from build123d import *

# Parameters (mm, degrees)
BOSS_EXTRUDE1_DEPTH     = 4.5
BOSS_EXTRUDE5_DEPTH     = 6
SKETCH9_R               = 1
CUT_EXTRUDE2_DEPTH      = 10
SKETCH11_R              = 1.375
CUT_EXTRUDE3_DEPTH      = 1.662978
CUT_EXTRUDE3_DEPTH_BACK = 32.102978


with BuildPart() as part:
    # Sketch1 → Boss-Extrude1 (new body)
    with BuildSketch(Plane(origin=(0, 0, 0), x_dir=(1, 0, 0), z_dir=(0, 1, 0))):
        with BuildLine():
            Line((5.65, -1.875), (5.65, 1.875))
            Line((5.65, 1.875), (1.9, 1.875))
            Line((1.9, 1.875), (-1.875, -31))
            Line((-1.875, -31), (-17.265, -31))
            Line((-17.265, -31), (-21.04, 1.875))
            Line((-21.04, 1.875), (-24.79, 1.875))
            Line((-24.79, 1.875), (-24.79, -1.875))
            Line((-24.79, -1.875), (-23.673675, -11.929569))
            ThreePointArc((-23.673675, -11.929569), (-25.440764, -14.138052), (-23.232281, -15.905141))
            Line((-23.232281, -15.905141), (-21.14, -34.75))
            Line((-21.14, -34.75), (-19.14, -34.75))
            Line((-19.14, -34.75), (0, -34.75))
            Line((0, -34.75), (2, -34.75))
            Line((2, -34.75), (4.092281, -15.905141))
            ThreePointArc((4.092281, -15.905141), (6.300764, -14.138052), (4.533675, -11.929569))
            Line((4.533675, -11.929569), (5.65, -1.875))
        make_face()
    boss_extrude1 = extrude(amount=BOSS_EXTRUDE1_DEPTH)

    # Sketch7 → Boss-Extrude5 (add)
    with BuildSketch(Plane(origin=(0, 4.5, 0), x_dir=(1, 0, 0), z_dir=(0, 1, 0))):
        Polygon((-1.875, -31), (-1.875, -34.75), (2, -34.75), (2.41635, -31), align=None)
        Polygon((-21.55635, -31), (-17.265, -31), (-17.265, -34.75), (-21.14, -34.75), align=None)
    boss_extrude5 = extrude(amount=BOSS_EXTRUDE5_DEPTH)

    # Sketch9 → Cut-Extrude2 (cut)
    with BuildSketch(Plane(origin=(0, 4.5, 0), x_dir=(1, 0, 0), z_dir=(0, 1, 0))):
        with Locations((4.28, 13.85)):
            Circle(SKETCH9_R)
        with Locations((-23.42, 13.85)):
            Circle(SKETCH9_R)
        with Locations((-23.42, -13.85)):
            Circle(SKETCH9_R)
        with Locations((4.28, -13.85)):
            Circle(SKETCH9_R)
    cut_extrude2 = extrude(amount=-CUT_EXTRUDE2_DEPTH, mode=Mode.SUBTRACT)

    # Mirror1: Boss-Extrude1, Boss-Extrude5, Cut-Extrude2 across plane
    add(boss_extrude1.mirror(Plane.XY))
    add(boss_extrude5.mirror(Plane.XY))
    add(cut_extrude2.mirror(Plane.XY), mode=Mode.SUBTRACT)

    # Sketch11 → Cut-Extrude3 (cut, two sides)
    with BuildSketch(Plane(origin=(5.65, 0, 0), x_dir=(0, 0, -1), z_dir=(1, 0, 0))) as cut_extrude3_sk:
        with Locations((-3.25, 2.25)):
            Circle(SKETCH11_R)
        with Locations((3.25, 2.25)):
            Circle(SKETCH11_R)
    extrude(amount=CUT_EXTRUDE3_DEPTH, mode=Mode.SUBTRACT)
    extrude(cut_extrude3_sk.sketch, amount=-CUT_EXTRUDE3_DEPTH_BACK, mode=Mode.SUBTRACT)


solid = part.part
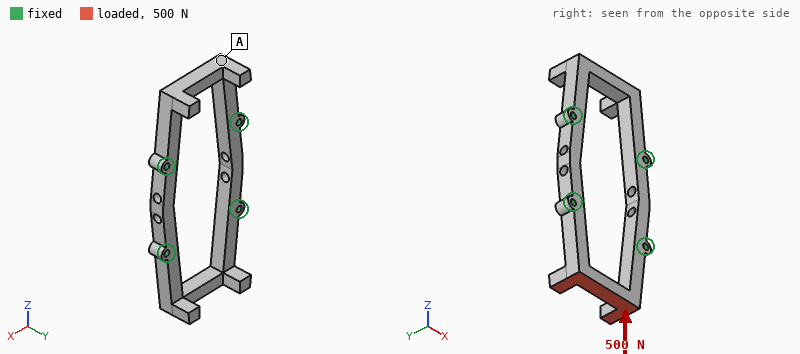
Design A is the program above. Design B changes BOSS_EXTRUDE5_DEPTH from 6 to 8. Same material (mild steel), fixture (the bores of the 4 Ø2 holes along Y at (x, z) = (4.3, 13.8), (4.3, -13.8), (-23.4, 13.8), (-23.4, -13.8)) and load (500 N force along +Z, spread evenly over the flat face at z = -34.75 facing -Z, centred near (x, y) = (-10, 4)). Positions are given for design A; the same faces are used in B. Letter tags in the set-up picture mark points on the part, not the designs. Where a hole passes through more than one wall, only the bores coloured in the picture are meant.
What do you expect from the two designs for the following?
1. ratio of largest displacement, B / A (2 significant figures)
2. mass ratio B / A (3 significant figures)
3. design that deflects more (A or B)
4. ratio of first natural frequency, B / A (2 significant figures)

1.6
1.04
B
0.94
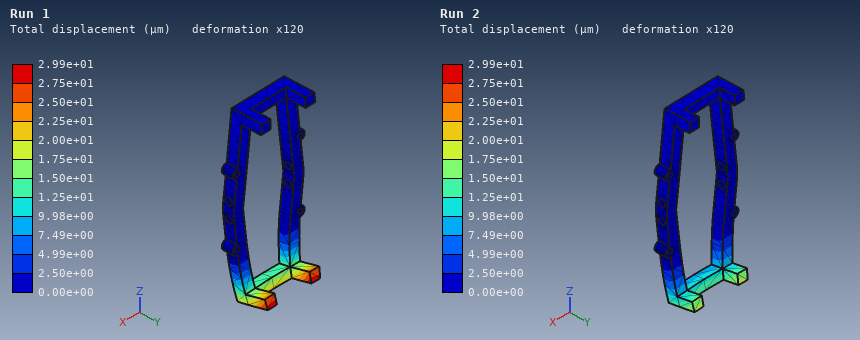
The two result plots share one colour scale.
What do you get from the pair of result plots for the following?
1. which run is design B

Run 1
